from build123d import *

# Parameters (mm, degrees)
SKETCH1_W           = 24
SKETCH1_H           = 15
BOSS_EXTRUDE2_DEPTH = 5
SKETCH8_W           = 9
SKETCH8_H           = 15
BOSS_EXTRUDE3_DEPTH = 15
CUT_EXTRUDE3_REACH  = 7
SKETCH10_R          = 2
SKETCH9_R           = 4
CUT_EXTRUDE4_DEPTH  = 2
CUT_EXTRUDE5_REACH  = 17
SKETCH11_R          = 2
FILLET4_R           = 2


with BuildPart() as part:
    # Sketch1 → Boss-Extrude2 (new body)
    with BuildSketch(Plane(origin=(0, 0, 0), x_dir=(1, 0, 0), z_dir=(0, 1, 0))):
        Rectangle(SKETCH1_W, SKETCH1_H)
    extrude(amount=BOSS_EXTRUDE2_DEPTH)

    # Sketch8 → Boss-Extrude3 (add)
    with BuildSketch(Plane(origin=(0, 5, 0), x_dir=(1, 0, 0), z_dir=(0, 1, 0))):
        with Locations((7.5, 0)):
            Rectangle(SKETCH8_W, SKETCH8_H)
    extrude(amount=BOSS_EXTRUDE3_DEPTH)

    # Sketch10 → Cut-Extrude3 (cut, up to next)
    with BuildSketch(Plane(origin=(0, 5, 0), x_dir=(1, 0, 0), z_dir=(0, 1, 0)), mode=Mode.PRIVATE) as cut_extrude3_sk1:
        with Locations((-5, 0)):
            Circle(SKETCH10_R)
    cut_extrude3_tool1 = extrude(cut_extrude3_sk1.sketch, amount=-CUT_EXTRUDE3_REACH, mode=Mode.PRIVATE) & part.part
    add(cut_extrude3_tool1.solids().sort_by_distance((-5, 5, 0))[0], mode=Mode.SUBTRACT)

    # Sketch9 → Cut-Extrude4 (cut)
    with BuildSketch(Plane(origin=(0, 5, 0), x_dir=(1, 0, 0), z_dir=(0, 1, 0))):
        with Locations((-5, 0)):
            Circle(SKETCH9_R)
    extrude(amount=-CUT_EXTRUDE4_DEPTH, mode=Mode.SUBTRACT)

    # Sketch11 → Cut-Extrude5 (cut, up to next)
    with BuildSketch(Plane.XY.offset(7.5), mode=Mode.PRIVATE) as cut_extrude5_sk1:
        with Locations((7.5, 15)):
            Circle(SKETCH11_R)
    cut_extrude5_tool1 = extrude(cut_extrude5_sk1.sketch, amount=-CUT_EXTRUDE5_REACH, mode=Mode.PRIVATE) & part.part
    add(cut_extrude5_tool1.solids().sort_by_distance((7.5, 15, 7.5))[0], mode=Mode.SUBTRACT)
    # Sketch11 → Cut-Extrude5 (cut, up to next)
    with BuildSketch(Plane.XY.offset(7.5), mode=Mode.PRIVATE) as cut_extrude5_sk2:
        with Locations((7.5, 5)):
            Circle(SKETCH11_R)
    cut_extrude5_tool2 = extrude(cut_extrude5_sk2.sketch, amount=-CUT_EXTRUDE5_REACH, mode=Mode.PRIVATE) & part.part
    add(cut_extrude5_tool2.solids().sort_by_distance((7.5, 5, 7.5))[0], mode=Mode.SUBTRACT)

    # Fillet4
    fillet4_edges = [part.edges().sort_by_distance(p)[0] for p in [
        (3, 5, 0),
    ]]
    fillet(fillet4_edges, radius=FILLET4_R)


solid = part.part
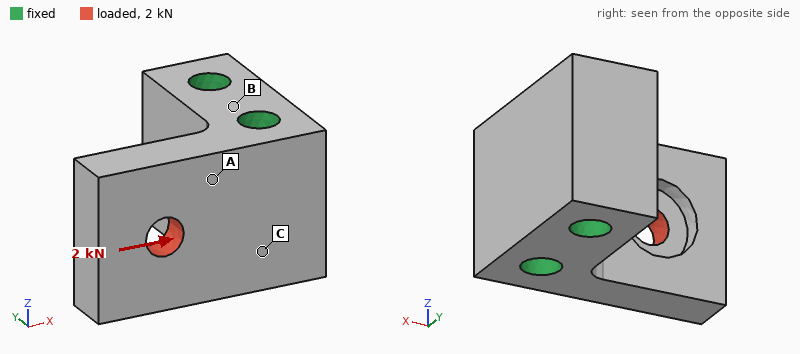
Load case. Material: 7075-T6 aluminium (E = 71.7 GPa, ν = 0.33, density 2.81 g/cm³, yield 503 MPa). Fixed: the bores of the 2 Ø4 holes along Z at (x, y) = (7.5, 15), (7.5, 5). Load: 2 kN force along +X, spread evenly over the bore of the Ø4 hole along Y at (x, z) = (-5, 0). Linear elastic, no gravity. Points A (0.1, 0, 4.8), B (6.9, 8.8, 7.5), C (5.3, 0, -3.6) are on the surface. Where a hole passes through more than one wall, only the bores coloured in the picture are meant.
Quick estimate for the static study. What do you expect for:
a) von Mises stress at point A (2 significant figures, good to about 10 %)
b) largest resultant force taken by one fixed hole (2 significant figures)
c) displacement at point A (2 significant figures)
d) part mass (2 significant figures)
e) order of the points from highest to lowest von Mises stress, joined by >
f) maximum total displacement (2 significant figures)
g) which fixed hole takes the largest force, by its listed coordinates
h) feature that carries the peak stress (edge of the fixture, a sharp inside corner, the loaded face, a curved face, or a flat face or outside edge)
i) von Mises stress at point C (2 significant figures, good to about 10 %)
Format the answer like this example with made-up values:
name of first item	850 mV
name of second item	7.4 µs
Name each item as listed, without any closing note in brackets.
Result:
von Mises stress at point A	54 MPa
largest resultant force taken by one fixed hole	2.2 kN
displacement at point A	8.3 µm
part mass	9.3 g
order of the points from highest to lowest von Mises stress, joined by >	A > C > B
maximum total displacement	31 µm
which fixed hole takes the largest force, by its listed coordinates	(7.5, 5)
feature that carries the peak stress	the loaded face
von Mises stress at point C	36 MPa
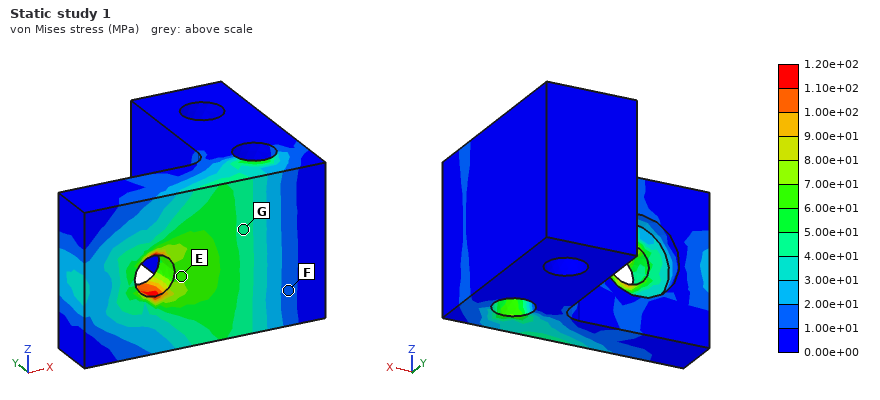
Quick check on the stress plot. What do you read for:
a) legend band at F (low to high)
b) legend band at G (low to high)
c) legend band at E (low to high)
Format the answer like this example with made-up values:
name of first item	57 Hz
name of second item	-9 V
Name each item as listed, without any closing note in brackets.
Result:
legend band at F	1.00e+01 to 2.00e+01 MPa
legend band at G	4.00e+01 to 5.00e+01 MPa
legend band at E	6.00e+01 to 7.00e+01 MPa
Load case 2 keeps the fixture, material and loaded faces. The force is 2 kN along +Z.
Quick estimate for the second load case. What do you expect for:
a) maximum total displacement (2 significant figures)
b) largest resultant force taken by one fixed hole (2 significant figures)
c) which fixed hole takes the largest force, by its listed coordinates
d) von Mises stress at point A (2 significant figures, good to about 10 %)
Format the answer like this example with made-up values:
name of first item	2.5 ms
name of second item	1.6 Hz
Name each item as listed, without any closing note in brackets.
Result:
maximum total displacement	39 µm
largest resultant force taken by one fixed hole	2.0 kN
which fixed hole takes the largest force, by its listed coordinates	(7.5, 5)
von Mises stress at point A	53 MPa
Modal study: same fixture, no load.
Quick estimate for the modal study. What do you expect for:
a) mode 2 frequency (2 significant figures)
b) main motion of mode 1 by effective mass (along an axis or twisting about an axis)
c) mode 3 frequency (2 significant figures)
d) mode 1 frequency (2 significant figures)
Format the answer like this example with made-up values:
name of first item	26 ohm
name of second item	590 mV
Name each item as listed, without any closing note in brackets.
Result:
mode 2 frequency	23 kHz
main motion of mode 1 by effective mass	along Y
mode 3 frequency	29 kHz
mode 1 frequency	14 kHz
